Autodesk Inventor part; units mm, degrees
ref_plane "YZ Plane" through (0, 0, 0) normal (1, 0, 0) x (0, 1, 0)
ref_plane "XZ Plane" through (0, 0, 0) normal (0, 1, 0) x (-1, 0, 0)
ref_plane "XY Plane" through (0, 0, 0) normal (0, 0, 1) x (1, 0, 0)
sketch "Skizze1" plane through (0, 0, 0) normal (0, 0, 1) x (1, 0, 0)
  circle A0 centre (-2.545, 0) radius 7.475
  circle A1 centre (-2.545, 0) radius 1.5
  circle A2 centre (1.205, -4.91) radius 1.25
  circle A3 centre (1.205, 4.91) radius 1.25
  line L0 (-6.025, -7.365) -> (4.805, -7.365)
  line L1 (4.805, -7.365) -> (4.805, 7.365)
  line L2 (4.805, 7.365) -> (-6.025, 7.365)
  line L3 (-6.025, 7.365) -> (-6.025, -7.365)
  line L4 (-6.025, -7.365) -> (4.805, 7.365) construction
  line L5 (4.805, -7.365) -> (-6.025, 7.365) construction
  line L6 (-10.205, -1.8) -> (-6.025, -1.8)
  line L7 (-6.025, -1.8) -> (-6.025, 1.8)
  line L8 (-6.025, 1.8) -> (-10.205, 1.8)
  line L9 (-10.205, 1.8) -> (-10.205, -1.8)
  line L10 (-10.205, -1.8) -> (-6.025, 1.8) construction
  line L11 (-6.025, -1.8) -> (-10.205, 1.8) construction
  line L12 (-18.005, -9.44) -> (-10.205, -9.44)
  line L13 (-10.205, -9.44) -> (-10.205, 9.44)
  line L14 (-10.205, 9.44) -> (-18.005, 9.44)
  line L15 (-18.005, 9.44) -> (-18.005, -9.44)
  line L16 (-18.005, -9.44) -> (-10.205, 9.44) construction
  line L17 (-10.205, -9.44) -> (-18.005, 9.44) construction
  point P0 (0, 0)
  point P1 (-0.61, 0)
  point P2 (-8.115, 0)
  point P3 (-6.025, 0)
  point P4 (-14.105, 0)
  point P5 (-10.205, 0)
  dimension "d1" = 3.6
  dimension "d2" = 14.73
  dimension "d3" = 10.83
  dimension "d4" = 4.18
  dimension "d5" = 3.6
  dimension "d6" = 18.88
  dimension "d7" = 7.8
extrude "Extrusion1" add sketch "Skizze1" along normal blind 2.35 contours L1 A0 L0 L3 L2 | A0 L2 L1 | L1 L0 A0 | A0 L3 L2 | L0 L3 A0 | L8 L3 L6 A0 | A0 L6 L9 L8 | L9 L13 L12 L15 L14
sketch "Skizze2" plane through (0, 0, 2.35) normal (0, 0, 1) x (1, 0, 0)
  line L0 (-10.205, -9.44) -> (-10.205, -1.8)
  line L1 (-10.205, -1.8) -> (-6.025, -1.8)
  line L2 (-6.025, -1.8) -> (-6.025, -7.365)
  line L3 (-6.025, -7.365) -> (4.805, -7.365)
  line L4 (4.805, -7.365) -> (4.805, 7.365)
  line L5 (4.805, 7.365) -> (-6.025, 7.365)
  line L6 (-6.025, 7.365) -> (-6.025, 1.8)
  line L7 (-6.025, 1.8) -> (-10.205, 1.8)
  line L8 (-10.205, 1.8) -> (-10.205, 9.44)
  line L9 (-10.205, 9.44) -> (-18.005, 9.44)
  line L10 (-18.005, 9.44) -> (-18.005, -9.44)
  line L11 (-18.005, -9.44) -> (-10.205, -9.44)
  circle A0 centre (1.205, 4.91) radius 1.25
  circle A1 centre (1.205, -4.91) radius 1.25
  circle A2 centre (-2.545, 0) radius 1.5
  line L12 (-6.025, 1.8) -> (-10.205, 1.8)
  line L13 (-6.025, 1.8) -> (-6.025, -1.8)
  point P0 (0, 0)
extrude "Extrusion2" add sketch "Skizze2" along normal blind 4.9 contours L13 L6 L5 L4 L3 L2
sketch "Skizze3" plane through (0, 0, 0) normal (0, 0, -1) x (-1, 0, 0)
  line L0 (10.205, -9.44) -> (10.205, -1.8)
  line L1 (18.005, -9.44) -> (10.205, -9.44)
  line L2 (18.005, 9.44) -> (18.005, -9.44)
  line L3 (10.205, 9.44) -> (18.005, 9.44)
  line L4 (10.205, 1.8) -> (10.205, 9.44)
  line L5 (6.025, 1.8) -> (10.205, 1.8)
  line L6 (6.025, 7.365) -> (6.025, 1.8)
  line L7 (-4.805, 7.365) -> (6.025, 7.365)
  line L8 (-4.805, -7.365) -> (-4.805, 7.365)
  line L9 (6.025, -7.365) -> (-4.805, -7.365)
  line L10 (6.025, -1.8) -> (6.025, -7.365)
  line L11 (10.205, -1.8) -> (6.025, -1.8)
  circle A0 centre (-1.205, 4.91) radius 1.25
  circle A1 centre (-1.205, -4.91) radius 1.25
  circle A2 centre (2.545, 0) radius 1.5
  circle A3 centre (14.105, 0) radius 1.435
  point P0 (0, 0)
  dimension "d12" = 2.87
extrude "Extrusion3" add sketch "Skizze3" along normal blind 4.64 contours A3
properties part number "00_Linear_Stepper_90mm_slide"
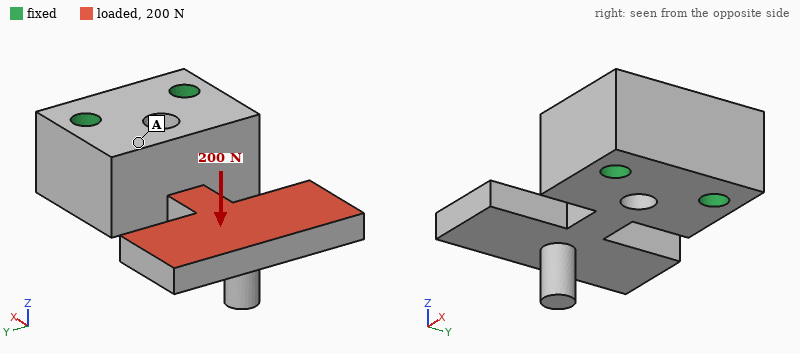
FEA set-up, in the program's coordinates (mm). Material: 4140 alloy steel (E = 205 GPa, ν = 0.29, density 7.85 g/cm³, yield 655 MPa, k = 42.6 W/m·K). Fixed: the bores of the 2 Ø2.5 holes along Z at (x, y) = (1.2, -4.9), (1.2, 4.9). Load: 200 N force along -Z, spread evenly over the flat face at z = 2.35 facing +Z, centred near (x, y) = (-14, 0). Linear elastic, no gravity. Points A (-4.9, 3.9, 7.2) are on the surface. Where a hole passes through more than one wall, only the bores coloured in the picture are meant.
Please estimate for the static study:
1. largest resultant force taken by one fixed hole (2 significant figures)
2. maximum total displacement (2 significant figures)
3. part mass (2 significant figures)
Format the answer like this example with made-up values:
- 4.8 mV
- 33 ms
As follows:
- 100 N
- 0.10 mm
- 11 g
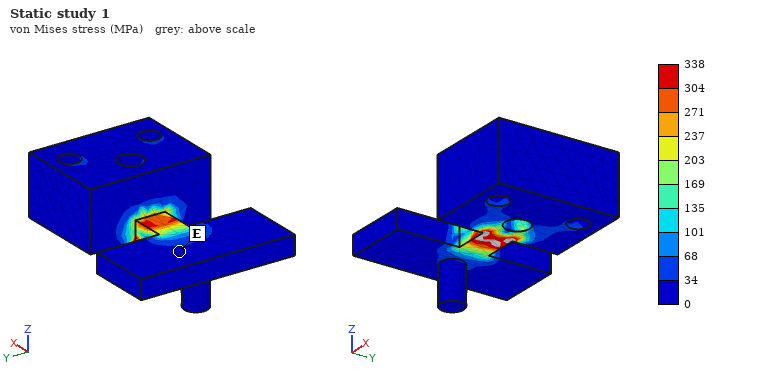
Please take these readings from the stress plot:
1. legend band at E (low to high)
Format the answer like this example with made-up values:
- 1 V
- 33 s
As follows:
- 0 to 34 MPa
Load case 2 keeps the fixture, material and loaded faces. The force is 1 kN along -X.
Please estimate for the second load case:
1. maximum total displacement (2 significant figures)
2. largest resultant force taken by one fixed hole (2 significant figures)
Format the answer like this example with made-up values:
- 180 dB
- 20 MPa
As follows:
- 89 µm
- 550 N
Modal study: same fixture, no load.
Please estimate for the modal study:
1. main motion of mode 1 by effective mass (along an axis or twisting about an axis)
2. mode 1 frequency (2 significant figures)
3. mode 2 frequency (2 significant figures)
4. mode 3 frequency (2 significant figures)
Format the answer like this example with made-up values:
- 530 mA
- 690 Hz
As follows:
- along Z
- 4700 Hz
- 5800 Hz
- 6000 Hz
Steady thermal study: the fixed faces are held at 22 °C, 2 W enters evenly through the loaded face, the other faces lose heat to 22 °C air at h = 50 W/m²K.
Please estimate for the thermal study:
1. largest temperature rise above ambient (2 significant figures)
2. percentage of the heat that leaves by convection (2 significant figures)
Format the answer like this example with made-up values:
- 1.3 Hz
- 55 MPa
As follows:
- 33 K
- 27 %
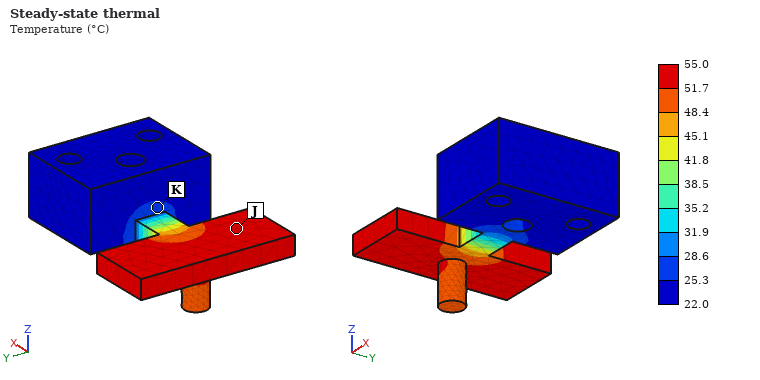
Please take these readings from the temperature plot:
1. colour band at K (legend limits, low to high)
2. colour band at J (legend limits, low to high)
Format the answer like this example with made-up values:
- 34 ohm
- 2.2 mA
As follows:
- 25.3 to 28.6 °C
- 51.7 to 55.0 °C
